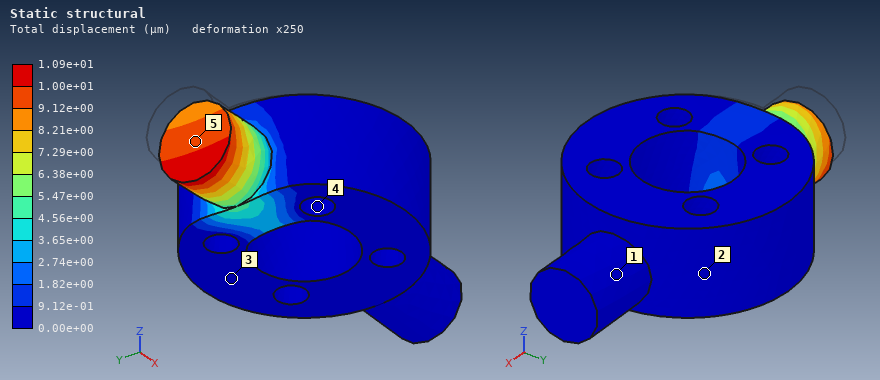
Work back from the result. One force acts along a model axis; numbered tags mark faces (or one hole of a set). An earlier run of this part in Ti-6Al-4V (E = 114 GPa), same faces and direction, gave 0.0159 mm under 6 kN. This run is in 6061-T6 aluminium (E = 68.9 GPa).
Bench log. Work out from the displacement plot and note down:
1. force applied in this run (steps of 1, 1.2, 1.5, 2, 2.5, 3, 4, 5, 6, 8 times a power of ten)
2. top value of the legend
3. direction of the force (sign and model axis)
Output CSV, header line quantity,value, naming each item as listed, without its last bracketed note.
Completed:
quantity,value
force applied in this run,2.5 kN
top value of the legend,1.09e+01 µm
direction of the force,+X
